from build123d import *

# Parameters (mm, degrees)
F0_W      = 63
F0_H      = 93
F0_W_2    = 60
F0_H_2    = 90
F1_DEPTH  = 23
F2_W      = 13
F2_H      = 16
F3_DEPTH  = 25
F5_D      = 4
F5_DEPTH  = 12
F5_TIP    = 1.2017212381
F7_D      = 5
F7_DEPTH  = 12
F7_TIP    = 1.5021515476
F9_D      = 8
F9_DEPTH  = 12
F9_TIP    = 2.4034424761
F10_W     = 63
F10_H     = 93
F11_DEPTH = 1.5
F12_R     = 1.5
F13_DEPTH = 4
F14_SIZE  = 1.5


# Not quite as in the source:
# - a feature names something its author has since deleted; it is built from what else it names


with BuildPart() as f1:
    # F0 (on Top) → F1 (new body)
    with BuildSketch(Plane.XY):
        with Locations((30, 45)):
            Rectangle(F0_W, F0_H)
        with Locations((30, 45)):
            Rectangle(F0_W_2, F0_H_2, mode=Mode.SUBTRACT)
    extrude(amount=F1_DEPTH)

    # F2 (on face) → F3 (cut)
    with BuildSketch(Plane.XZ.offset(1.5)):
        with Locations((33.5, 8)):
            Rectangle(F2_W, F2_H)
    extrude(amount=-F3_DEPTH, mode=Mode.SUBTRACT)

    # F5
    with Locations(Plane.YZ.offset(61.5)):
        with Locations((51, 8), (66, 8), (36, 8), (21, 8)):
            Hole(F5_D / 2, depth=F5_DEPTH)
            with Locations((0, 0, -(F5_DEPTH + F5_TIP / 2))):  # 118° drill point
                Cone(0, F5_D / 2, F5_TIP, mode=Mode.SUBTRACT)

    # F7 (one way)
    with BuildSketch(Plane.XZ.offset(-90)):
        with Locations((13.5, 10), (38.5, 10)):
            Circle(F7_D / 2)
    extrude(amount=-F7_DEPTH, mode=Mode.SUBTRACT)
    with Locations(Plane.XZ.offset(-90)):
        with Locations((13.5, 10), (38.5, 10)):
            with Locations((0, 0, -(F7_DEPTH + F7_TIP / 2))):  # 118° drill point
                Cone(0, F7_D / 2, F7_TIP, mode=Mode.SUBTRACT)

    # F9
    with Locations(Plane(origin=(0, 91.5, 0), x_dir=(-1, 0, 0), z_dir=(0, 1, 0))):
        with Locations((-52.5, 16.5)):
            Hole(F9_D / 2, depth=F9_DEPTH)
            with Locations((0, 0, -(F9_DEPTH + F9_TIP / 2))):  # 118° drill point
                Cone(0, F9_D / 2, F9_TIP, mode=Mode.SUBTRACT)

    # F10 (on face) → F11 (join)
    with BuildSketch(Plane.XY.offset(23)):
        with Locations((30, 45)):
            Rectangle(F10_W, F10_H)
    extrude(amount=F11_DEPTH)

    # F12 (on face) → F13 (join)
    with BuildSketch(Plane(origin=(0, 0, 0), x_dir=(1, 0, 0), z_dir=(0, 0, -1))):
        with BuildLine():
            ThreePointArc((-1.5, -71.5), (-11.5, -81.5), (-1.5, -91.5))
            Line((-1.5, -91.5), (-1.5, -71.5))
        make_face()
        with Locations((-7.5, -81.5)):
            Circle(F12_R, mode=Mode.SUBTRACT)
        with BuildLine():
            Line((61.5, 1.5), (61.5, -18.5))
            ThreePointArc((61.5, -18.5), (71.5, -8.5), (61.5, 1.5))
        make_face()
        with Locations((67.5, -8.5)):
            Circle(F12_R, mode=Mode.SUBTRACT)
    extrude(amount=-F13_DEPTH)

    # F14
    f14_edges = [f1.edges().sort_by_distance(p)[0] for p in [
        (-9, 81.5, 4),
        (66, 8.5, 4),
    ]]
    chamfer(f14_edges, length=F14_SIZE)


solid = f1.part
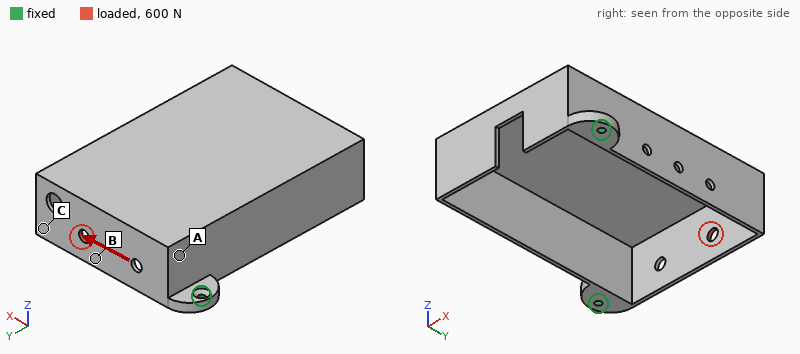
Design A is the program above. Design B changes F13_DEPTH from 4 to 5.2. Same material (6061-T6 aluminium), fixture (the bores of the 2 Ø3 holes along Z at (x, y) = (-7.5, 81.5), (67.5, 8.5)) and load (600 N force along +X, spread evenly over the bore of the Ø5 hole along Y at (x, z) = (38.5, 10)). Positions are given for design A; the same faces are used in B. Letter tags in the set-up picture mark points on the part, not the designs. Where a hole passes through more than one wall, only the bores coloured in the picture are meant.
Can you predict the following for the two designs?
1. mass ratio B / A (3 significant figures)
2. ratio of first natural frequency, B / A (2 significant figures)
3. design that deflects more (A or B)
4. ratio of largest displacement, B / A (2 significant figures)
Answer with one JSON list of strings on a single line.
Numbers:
["1.02", "1.4", "A", "0.53"]
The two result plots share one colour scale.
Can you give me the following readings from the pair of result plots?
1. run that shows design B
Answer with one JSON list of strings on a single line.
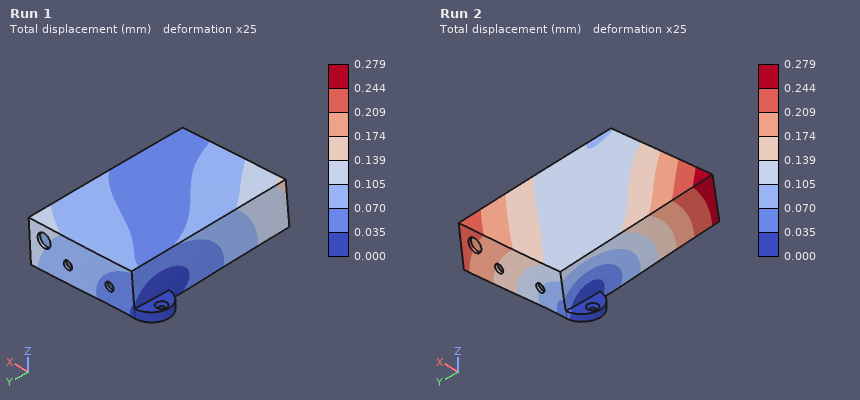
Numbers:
["Run 1"]
